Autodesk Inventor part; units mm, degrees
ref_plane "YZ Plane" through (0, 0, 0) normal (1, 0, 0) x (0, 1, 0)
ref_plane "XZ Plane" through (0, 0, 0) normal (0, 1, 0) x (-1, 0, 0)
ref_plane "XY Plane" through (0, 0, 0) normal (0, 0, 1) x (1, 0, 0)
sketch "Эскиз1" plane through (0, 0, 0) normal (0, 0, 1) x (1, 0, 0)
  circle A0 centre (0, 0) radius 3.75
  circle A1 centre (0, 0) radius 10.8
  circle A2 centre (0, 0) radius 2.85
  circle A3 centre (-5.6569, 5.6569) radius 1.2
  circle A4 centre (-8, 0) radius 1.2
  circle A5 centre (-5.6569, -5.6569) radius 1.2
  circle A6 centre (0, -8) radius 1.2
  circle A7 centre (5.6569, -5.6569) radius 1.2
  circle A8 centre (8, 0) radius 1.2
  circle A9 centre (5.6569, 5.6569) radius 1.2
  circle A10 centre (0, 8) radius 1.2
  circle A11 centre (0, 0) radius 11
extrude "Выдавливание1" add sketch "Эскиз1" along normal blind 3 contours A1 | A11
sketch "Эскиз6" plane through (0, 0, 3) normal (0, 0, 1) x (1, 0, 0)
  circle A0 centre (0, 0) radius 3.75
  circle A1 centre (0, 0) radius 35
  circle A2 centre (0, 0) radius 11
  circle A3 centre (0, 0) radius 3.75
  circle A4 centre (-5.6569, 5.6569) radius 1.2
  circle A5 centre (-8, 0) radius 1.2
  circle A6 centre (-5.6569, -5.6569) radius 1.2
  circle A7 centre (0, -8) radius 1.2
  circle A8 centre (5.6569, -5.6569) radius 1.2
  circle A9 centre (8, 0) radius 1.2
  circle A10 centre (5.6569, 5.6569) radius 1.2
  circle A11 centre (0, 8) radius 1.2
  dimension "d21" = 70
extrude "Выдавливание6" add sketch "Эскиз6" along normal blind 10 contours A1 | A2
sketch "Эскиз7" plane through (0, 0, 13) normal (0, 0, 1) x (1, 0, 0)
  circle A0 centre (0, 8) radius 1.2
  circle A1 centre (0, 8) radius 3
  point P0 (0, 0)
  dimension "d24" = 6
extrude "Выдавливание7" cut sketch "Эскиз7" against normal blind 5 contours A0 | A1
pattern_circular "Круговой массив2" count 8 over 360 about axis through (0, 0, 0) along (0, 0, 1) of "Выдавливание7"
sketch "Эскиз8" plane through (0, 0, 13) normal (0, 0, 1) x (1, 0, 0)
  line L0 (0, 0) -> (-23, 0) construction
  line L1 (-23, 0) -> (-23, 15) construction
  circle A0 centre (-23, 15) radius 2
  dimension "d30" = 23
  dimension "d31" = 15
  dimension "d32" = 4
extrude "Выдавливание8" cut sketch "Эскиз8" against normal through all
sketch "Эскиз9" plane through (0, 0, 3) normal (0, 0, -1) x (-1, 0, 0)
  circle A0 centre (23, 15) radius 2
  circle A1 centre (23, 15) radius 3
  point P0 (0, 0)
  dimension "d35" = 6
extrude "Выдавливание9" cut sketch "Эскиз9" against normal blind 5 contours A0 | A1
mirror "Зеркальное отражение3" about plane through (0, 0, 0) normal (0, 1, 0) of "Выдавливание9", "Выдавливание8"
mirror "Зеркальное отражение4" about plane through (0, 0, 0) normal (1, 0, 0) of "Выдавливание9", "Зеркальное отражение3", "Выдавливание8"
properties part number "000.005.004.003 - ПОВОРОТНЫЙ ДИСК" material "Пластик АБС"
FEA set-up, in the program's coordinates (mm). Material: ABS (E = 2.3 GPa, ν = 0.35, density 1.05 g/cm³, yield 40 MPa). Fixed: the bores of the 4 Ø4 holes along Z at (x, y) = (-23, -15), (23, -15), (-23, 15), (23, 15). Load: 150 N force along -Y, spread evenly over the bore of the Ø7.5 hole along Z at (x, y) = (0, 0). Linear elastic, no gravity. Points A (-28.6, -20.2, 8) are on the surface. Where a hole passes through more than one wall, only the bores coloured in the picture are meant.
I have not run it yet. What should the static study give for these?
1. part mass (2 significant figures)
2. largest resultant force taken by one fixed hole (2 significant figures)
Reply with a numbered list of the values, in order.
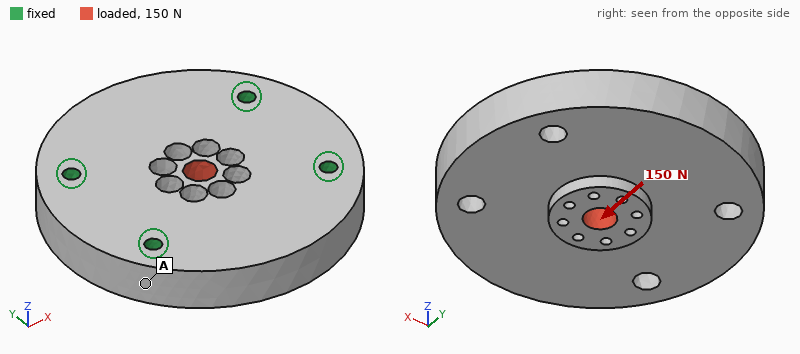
1. 39 g
2. 40 N
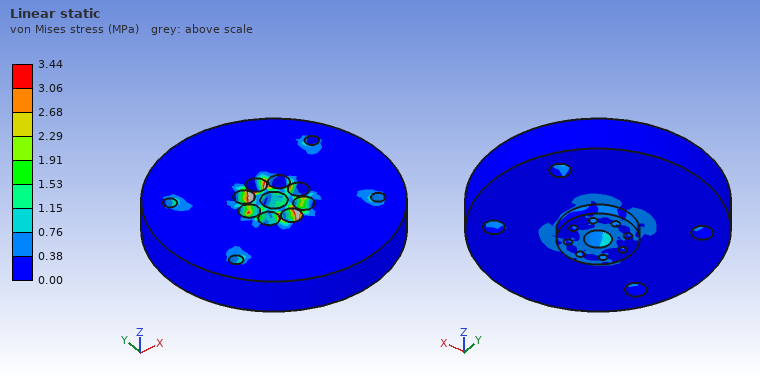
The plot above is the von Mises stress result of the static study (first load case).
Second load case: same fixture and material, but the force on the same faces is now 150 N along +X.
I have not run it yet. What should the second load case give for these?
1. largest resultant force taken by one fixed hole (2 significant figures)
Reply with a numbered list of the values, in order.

1. 39 N
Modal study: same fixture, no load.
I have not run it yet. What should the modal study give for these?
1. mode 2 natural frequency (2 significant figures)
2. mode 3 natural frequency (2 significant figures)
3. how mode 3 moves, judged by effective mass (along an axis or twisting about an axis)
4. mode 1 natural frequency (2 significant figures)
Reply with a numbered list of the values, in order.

1. 3200 Hz
2. 5100 Hz
3. along Z
4. 3100 Hz
